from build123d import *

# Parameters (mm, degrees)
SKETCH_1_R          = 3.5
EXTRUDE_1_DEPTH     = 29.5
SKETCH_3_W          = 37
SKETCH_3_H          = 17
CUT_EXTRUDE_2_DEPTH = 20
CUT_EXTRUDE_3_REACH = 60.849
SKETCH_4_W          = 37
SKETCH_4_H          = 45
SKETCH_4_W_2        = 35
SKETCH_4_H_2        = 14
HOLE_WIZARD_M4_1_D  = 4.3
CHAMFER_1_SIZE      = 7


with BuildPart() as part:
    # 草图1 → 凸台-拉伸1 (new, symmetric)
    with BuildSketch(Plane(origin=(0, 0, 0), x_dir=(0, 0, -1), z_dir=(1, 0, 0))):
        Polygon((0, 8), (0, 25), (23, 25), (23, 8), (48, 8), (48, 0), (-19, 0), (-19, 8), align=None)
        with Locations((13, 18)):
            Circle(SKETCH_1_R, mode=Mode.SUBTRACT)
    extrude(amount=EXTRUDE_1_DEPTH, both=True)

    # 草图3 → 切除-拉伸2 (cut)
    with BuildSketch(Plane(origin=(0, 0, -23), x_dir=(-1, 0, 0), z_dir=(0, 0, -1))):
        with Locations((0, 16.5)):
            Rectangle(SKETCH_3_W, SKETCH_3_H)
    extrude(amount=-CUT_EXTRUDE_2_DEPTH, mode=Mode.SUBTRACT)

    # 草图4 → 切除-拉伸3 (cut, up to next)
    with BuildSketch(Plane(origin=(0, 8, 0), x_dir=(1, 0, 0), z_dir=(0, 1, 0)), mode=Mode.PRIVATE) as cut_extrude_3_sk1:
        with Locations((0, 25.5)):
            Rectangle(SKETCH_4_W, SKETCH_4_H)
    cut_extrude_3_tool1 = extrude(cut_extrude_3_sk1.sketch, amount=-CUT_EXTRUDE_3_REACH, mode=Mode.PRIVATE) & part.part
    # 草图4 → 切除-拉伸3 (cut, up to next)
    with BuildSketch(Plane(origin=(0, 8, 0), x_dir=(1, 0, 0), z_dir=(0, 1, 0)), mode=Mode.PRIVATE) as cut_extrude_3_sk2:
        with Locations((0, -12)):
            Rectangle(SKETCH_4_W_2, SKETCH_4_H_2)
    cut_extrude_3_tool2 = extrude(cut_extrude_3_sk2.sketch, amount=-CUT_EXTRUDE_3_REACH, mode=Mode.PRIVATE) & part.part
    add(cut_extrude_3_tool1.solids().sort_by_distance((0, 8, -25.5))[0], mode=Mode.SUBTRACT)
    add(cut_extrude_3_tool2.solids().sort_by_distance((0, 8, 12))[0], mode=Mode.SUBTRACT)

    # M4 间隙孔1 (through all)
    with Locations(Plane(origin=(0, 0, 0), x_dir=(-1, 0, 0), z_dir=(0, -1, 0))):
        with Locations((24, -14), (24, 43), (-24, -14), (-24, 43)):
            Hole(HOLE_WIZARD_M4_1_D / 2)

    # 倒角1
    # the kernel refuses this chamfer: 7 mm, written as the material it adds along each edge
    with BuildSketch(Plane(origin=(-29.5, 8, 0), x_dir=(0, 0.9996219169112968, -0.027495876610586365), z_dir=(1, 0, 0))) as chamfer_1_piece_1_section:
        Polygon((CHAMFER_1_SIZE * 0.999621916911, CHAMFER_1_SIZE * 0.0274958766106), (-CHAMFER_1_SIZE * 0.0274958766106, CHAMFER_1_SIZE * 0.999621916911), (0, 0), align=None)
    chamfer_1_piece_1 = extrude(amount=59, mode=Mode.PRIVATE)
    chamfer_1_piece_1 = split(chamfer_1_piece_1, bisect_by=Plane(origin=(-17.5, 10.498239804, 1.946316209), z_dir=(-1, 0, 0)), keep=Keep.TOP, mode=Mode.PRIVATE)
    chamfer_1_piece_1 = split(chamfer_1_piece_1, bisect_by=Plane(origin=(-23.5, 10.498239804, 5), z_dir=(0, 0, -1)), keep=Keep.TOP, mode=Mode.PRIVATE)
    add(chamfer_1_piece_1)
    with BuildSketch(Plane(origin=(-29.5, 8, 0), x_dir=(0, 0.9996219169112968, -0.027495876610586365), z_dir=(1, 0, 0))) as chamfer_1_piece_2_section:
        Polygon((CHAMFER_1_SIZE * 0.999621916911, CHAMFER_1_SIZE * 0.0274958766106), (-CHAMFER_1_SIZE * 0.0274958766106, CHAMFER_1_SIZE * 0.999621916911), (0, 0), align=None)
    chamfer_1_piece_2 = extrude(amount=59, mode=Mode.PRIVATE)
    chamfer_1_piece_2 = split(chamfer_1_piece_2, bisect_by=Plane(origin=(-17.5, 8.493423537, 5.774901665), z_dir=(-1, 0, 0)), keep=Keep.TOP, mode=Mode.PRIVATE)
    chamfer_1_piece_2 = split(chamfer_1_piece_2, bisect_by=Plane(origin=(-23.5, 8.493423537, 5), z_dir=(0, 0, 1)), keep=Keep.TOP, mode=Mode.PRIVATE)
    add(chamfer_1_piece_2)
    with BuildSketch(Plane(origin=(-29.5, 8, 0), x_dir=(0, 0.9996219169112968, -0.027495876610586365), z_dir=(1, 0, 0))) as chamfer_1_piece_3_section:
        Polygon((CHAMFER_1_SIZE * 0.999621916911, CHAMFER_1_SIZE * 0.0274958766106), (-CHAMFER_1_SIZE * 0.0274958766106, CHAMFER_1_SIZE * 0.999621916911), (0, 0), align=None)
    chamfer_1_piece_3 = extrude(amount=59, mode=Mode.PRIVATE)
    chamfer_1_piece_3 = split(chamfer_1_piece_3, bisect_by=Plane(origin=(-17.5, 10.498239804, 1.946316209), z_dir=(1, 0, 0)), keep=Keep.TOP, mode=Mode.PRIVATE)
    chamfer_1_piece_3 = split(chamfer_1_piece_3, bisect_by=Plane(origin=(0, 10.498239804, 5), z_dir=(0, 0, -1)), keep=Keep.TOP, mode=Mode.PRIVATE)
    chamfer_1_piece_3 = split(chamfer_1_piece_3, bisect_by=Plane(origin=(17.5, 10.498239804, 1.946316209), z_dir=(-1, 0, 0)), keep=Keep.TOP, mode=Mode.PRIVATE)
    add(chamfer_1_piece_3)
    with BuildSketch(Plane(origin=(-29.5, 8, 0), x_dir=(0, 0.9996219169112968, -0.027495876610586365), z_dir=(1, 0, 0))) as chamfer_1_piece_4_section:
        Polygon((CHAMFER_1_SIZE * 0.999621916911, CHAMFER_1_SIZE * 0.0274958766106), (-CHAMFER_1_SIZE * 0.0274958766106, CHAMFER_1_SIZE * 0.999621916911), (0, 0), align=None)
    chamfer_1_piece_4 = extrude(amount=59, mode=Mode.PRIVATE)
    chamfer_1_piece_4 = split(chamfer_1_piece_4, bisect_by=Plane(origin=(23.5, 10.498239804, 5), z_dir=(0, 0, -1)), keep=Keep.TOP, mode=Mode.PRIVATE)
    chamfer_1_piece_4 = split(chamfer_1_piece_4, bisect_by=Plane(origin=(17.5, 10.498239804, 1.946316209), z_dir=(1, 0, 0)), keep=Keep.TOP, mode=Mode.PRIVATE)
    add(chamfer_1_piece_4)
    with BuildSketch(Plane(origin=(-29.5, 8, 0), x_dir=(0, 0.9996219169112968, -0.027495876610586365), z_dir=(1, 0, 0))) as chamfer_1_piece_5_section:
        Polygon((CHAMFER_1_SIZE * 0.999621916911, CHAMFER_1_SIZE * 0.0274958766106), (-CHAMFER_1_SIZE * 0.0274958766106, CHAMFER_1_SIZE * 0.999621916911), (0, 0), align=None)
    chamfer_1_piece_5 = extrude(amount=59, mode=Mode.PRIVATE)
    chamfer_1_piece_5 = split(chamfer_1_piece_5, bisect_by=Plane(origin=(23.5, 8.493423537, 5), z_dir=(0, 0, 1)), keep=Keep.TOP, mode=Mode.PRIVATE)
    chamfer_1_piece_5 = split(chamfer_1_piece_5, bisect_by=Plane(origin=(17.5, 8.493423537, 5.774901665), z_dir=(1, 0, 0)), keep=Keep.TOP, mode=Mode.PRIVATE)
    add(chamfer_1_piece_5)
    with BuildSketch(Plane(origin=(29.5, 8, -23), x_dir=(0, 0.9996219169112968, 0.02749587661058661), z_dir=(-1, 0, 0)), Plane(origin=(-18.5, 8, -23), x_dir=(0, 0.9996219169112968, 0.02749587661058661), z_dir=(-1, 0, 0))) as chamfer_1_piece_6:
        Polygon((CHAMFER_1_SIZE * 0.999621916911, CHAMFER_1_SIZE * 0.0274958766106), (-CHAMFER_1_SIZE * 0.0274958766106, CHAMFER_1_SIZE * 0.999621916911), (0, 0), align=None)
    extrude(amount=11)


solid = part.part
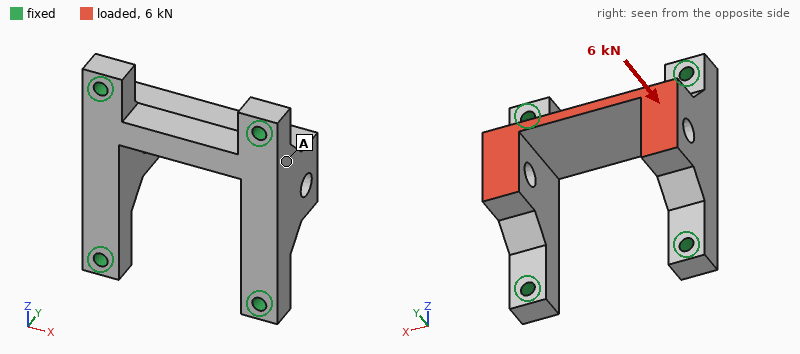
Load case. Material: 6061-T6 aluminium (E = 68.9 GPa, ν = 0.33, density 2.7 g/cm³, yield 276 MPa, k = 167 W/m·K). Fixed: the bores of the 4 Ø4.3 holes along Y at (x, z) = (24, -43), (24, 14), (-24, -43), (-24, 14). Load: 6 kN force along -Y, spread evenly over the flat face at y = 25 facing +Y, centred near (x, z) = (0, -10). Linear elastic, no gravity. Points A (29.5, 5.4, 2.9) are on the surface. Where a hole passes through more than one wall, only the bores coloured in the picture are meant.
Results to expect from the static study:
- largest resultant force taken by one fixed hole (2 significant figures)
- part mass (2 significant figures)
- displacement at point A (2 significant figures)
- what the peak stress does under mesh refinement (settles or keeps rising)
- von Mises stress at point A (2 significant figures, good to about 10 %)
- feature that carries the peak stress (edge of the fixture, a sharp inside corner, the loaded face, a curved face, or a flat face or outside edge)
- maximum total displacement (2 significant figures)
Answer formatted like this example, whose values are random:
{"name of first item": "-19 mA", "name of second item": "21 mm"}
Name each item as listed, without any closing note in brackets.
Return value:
{"largest resultant force taken by one fixed hole": "2.0 kN", "part mass": "69 g", "displacement at point A": "15 µm", "what the peak stress does under mesh refinement": "keeps rising", "von Mises stress at point A": "23 MPa", "feature that carries the peak stress": "edge of the fixture", "maximum total displacement": "34 µm"}
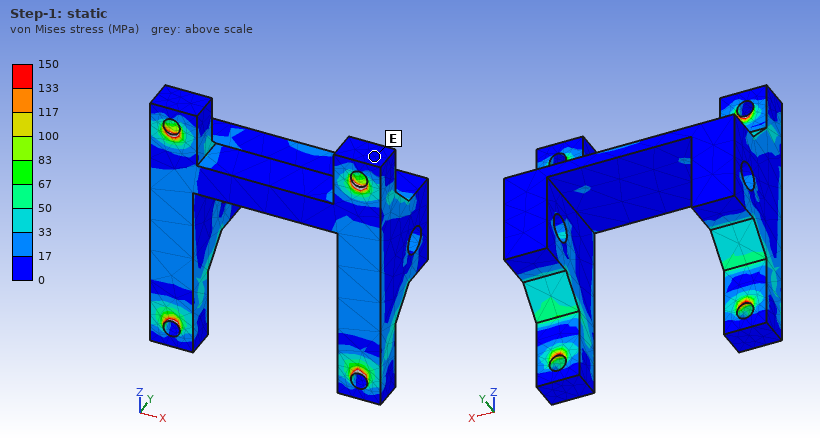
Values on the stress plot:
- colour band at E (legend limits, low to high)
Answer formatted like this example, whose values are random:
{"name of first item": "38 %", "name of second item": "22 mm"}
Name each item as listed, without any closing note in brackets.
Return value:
{"colour band at E": "0 to 17 MPa"}
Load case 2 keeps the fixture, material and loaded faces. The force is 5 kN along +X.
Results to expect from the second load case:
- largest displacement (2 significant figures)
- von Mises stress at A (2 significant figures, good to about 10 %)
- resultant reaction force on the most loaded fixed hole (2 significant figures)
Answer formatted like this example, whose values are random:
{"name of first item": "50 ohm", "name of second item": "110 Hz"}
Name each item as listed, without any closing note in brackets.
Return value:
{"largest displacement": "0.10 mm", "von Mises stress at A": "43 MPa", "resultant reaction force on the most loaded fixed hole": "2.6 kN"}
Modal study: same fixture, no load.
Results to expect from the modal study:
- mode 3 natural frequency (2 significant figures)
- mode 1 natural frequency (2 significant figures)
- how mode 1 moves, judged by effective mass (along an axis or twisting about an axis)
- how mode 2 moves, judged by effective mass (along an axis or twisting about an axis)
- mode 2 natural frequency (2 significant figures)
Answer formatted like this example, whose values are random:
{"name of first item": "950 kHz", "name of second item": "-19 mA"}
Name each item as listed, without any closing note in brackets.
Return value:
{"mode 3 natural frequency": "12 kHz", "mode 1 natural frequency": "8900 Hz", "how mode 1 moves, judged by effective mass": "along X", "how mode 2 moves, judged by effective mass": "along Y", "mode 2 natural frequency": "10 kHz"}
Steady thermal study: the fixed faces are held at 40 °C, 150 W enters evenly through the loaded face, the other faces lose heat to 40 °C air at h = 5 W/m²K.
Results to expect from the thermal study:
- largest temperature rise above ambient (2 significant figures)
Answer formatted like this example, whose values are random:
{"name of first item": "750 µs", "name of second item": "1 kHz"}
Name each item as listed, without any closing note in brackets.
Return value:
{"largest temperature rise above ambient": "66 K"}
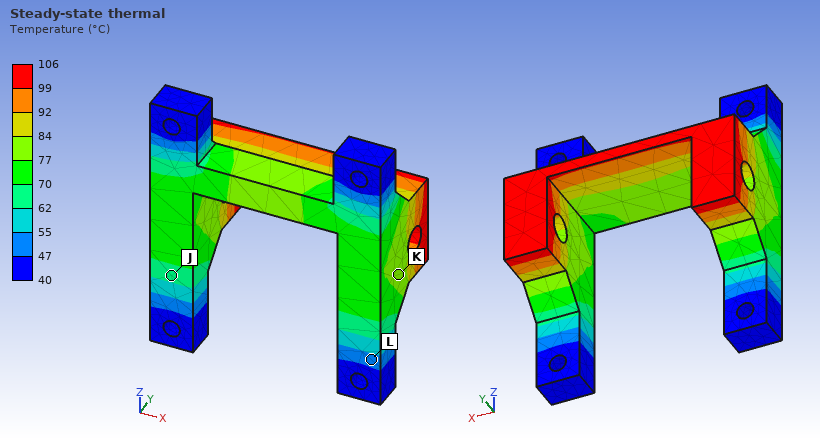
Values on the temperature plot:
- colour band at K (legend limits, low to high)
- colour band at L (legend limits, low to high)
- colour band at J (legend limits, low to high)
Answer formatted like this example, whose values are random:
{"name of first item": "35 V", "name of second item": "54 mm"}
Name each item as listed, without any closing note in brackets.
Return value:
{"colour band at K": "77 to 84 °C", "colour band at L": "47 to 55 °C", "colour band at J": "62 to 70 °C"}
